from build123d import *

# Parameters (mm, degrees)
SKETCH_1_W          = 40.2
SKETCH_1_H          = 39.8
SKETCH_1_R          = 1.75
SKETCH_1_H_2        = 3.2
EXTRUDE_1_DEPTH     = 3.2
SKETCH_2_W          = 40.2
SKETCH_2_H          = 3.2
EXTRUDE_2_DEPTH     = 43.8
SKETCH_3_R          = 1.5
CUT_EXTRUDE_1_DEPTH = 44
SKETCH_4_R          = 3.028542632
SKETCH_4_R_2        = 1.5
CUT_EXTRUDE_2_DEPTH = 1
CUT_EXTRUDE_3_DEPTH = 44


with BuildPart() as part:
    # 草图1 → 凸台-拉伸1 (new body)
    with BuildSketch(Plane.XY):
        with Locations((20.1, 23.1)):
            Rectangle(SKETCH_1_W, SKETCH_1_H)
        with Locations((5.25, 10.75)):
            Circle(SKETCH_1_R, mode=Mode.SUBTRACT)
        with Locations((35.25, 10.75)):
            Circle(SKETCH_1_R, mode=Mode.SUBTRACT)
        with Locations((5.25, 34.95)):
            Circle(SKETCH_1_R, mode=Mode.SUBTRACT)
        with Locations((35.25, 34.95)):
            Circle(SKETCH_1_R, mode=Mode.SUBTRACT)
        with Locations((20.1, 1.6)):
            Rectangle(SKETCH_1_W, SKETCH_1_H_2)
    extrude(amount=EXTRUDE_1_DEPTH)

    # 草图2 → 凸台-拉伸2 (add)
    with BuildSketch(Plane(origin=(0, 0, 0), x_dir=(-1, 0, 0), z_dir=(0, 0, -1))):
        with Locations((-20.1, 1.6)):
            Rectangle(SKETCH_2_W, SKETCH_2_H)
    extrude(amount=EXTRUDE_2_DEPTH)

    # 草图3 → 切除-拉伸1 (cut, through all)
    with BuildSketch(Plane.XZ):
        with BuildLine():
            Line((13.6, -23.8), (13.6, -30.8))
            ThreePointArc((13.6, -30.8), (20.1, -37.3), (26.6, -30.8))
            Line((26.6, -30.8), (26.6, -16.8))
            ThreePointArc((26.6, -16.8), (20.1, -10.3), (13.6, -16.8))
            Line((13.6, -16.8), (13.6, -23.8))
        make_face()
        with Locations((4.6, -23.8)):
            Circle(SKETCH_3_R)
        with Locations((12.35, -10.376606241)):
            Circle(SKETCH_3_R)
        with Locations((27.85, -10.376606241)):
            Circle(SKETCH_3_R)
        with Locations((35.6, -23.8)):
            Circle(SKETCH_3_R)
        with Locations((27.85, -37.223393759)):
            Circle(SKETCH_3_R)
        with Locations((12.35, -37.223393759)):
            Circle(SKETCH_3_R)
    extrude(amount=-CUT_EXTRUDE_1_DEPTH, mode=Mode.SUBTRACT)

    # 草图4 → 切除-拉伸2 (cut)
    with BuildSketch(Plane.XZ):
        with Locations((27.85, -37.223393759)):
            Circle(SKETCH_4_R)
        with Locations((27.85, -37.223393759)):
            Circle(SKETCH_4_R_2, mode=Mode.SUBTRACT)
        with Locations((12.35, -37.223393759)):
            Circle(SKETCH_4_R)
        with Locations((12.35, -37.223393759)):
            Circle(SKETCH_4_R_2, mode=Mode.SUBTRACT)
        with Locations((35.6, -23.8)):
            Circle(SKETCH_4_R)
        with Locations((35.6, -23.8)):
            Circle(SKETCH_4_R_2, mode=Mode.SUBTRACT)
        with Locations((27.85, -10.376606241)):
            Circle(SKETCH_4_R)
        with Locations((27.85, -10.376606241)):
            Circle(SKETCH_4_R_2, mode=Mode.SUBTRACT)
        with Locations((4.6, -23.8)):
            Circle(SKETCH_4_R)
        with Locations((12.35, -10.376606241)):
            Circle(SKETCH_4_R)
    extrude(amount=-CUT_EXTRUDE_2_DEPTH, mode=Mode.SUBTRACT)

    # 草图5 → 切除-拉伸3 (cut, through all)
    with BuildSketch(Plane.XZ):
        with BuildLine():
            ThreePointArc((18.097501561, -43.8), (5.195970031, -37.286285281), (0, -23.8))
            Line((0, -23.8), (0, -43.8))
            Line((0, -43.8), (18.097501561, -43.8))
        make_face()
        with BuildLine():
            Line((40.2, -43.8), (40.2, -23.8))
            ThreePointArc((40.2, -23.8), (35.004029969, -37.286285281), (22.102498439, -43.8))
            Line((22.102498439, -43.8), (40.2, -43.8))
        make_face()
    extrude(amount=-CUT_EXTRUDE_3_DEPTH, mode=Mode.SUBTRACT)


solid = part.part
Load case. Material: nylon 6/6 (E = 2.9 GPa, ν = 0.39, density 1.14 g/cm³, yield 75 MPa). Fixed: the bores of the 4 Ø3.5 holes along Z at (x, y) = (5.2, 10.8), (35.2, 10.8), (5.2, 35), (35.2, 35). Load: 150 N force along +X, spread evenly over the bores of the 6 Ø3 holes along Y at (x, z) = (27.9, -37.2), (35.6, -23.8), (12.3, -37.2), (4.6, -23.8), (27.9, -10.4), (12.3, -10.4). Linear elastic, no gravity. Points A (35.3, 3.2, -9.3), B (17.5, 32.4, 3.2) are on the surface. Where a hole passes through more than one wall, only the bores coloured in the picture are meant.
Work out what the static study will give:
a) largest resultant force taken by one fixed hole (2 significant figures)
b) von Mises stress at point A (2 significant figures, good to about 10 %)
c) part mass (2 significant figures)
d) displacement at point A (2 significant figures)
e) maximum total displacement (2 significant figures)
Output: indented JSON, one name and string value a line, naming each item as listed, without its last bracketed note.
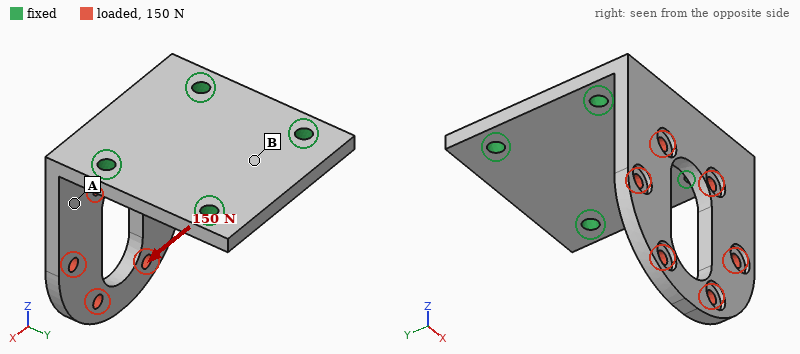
{
  "largest resultant force taken by one fixed hole": "150 N",
  "von Mises stress at point A": "7.2 MPa",
  "part mass": "11 g",
  "displacement at point A": "0.29 mm",
  "maximum total displacement": "0.72 mm"
}
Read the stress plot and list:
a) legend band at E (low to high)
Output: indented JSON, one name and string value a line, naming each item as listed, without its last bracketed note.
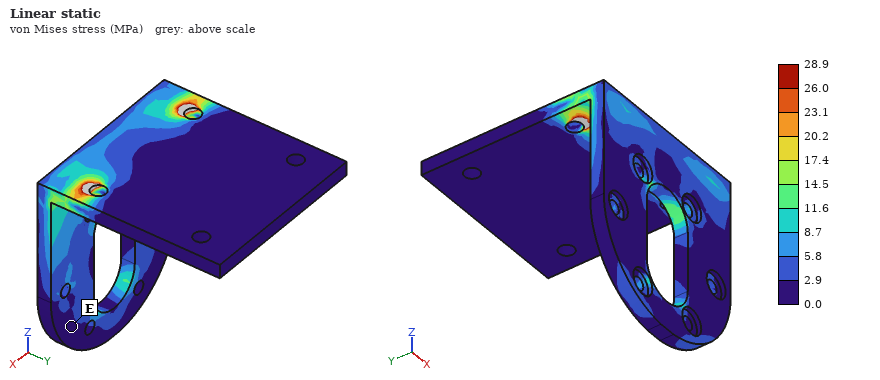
{
  "legend band at E": "0.0 to 2.9 MPa"
}
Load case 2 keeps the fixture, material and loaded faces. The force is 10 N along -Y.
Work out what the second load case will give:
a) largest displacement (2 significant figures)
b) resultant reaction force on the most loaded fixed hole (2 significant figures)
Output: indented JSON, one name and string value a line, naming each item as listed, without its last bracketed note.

{
  "largest displacement": "0.79 mm",
  "resultant reaction force on the most loaded fixed hole": "4.0 N"
}
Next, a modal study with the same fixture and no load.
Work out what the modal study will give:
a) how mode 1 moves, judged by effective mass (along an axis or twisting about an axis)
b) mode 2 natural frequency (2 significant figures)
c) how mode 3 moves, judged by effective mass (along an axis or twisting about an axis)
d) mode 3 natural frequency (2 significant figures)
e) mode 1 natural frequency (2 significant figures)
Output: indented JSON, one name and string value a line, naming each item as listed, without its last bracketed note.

{
  "how mode 1 moves, judged by effective mass": "along Y",
  "mode 2 natural frequency": "1000 Hz",
  "how mode 3 moves, judged by effective mass": "along X",
  "mode 3 natural frequency": "1600 Hz",
  "mode 1 natural frequency": "400 Hz"
}
